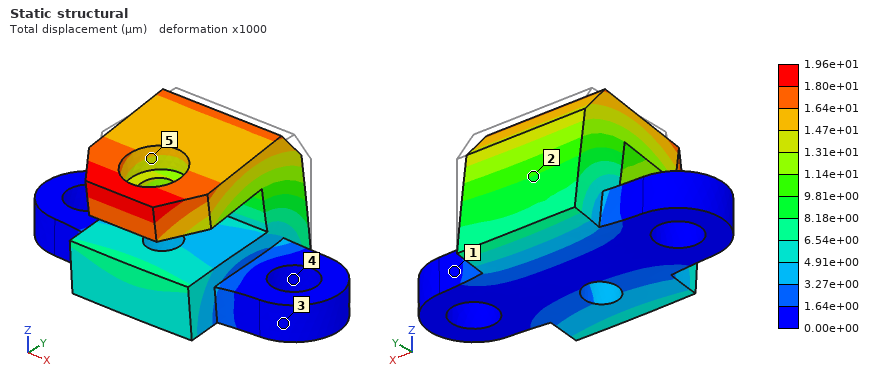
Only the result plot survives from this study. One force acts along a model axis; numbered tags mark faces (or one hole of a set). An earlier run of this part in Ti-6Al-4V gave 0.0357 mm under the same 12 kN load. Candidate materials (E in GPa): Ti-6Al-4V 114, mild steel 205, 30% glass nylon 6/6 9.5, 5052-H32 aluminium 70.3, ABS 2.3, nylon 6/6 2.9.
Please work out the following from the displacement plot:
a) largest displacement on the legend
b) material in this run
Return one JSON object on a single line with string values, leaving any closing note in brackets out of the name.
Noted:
{"largest displacement on the legend": "1.96e+01 µm", "material in this run": "mild steel"}
